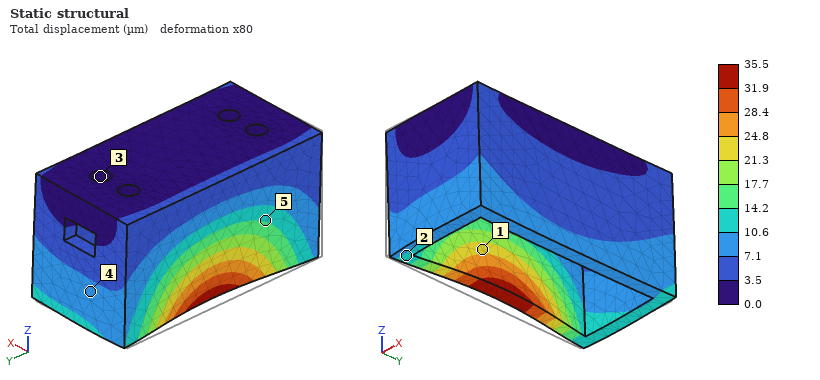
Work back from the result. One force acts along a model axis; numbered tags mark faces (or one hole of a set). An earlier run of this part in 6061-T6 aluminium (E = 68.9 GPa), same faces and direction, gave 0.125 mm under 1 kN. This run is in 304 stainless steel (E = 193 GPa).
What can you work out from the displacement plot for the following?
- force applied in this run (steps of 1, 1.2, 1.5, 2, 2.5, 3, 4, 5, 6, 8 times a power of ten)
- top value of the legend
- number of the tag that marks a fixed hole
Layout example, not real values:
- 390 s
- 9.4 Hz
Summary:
- 800 N
- 35.5 µm
- 3
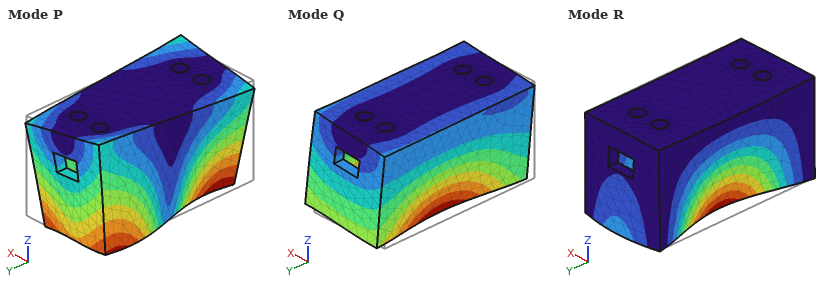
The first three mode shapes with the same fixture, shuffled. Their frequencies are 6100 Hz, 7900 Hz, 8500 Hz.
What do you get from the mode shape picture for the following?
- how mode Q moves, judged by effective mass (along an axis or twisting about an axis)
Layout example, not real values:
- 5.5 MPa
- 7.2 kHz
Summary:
- along X
